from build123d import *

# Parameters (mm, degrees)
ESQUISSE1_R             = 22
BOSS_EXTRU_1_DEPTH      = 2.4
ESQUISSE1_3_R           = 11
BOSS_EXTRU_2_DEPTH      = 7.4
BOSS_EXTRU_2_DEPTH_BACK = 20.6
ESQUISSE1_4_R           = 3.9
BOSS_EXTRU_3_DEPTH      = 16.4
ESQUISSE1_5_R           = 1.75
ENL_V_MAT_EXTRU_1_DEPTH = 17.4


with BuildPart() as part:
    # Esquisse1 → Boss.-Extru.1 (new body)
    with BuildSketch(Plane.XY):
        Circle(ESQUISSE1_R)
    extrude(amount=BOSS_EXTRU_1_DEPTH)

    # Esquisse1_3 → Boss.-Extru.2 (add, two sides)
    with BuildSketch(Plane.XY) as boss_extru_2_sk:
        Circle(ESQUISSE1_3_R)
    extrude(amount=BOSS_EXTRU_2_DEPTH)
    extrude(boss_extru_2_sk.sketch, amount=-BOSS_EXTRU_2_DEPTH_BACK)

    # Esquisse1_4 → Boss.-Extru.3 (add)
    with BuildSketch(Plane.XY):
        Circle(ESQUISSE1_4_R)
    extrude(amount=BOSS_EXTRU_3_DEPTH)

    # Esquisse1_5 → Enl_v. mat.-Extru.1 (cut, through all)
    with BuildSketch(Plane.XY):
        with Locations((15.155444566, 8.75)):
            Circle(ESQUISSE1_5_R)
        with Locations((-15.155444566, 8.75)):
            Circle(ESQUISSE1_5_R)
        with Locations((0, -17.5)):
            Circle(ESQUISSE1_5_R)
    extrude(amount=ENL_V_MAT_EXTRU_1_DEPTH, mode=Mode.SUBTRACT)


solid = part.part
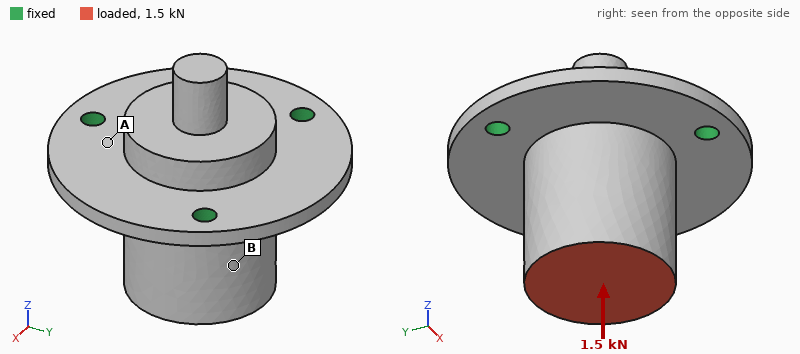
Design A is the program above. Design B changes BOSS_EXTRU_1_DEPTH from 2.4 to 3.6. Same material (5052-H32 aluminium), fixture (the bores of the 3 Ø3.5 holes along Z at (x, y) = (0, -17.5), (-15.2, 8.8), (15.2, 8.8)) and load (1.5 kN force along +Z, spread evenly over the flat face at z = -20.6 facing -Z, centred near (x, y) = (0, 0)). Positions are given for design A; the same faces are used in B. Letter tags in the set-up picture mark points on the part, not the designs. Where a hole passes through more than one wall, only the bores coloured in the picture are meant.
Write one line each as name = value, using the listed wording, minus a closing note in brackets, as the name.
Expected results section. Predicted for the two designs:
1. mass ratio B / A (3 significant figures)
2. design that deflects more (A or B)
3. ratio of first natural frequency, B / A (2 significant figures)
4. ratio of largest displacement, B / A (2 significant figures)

mass ratio B / A = 1.10
design that deflects more = A
ratio of first natural frequency, B / A = 1.4
ratio of largest displacement, B / A = 0.49
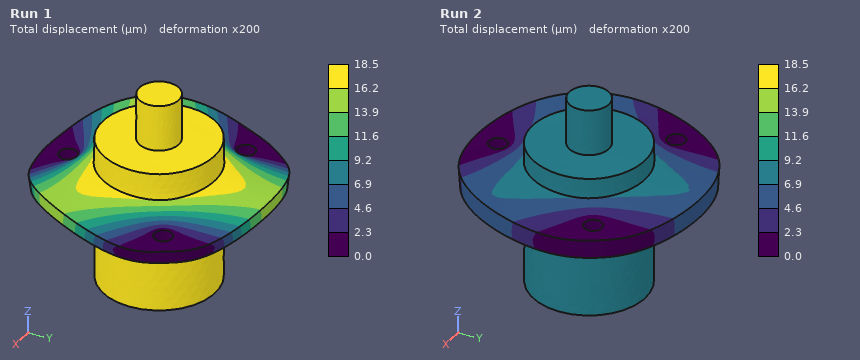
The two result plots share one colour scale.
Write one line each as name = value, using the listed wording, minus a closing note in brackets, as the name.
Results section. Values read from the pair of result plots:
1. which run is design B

which run is design B = Run 2
